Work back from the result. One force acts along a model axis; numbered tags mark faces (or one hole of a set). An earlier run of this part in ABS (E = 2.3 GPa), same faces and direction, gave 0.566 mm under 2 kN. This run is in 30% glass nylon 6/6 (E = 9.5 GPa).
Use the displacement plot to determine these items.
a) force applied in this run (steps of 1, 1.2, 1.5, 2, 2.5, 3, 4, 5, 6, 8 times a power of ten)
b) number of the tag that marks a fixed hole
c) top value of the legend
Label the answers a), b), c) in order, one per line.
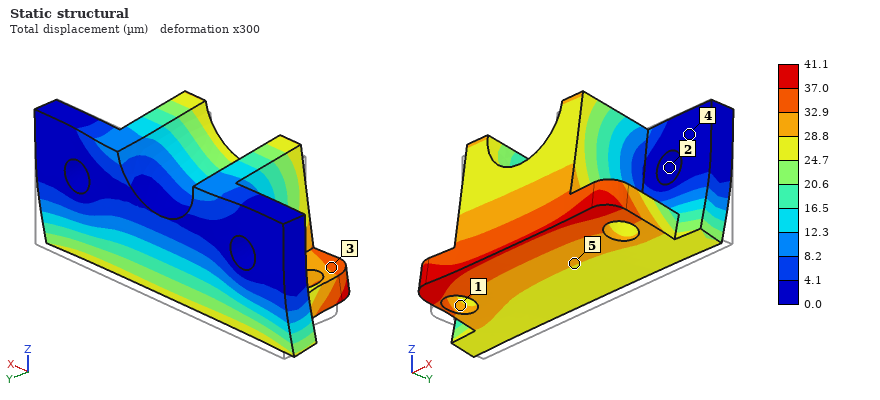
a) 600 N
b) 2
c) 41.1 µm
